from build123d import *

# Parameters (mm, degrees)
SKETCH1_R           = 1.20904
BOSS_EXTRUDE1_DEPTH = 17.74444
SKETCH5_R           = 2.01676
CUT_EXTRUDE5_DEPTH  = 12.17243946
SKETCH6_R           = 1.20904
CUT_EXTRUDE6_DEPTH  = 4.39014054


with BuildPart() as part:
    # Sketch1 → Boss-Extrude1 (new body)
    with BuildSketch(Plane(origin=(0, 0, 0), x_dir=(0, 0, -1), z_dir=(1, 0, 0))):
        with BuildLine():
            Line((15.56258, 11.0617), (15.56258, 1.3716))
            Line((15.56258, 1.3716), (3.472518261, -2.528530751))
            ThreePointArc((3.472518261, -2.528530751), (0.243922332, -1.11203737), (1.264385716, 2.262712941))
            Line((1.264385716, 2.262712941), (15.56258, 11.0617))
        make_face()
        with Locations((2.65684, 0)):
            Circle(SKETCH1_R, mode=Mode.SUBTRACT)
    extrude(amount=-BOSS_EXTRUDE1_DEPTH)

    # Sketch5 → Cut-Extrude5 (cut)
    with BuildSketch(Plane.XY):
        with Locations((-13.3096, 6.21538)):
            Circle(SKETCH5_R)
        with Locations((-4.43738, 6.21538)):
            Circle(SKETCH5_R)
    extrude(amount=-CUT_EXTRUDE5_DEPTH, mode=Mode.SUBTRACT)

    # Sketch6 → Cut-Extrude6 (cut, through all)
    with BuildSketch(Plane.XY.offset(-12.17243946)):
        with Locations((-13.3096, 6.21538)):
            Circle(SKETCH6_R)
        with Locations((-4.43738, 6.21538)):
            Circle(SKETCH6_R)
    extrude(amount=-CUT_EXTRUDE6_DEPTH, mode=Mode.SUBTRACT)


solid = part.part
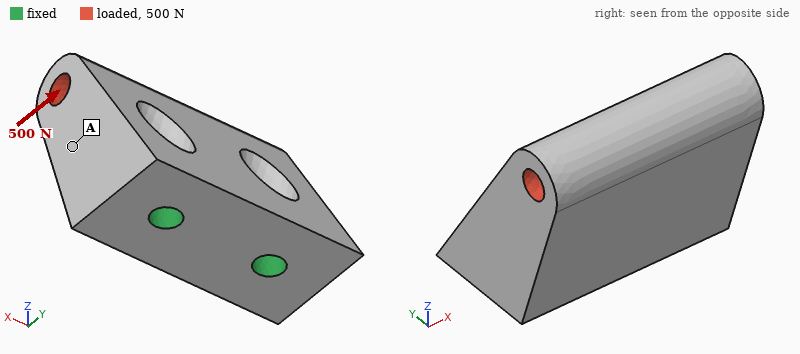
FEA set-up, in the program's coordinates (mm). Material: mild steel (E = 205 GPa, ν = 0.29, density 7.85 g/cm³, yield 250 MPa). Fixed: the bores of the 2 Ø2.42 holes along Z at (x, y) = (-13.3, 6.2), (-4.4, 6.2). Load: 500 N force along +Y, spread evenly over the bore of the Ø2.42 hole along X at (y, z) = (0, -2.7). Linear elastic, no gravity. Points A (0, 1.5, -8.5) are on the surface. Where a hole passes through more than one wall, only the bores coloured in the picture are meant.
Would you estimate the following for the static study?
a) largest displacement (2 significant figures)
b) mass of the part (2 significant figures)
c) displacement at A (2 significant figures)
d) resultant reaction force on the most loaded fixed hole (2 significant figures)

13 µm
14 g
4.8 µm
250 N
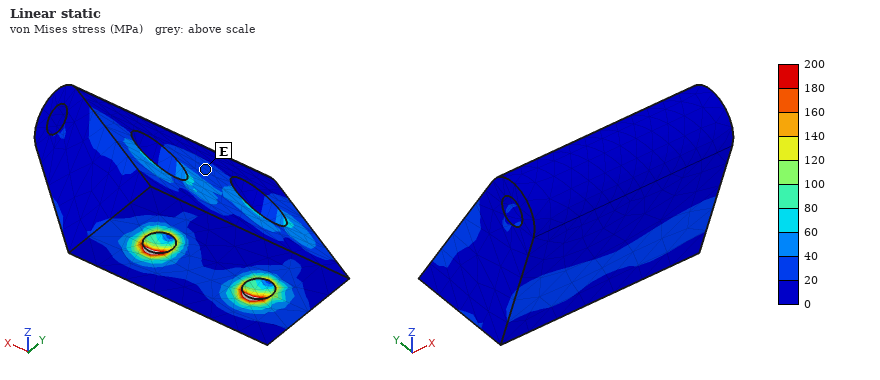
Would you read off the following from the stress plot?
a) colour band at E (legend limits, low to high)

20 to 40 MPa
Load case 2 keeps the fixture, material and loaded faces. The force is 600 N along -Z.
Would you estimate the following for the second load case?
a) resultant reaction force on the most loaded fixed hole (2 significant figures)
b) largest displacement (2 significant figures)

300 N
8.1 µm
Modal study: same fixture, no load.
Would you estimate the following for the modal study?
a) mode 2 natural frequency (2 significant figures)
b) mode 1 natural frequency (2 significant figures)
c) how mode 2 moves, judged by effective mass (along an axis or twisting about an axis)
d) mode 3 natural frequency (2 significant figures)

27 kHz
15 kHz
along X
35 kHz
